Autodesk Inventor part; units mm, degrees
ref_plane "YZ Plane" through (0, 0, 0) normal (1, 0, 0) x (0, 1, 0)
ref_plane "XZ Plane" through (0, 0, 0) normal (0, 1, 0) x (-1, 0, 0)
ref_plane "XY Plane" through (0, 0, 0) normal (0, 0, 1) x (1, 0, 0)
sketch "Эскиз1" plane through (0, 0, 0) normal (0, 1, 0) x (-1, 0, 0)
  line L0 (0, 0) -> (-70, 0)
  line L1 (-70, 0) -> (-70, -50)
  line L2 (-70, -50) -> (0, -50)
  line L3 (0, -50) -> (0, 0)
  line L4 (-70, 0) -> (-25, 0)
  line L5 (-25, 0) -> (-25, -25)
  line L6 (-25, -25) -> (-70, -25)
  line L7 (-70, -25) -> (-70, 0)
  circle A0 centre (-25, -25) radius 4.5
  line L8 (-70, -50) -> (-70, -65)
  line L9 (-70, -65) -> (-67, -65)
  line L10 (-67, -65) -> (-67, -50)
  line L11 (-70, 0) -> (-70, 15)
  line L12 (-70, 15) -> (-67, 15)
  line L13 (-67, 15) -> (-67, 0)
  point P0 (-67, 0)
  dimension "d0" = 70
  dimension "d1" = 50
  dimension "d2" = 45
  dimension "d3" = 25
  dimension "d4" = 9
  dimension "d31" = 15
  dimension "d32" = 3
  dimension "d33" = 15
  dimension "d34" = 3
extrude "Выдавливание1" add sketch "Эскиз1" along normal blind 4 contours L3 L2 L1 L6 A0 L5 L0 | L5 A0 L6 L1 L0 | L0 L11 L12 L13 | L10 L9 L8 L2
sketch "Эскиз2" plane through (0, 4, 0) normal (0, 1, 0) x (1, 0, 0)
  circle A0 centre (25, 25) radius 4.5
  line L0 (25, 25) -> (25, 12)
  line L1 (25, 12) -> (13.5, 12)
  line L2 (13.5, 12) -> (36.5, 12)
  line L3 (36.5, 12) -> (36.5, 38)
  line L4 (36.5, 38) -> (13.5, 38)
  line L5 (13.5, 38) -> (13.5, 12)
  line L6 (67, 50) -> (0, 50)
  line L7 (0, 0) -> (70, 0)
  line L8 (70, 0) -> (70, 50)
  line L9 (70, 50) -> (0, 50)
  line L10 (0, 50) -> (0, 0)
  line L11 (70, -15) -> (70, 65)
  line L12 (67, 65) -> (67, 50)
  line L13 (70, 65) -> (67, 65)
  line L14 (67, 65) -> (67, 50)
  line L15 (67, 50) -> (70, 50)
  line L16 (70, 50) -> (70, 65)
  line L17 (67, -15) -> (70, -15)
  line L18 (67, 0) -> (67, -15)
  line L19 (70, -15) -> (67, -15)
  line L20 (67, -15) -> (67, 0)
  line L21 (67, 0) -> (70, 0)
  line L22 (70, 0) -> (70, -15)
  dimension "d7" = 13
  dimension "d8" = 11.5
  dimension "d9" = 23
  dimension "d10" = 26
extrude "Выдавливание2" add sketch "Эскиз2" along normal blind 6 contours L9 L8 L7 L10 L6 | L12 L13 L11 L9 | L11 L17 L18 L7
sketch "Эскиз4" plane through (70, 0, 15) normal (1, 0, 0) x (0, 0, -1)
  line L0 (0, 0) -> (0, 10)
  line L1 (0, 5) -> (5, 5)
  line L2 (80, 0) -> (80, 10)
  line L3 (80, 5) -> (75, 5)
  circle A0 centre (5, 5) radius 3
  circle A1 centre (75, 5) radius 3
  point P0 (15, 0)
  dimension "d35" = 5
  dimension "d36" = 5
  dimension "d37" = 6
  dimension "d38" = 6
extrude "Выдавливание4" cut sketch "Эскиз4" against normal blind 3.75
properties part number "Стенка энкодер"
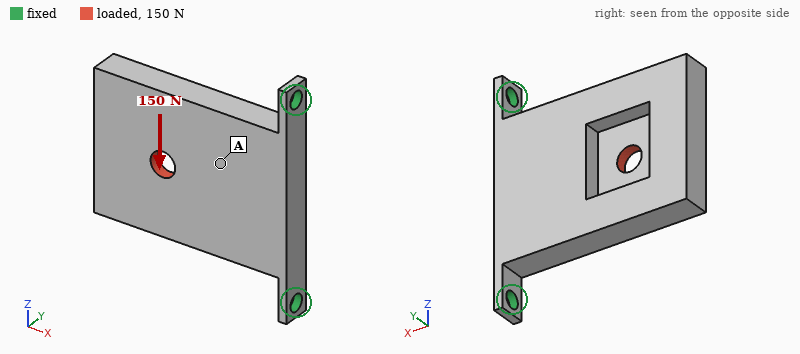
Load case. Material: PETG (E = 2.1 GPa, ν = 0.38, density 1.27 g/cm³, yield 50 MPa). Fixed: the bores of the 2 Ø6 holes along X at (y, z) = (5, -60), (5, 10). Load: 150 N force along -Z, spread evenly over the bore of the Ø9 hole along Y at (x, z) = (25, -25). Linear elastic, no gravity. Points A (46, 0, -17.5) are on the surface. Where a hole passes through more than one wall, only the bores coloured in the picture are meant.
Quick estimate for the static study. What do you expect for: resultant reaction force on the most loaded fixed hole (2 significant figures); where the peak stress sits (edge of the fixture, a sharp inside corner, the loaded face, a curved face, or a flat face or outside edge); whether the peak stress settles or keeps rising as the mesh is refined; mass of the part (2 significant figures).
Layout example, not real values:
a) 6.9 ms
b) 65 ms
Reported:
a) 140 N
b) edge of the fixture
c) keeps rising
d) 40 g
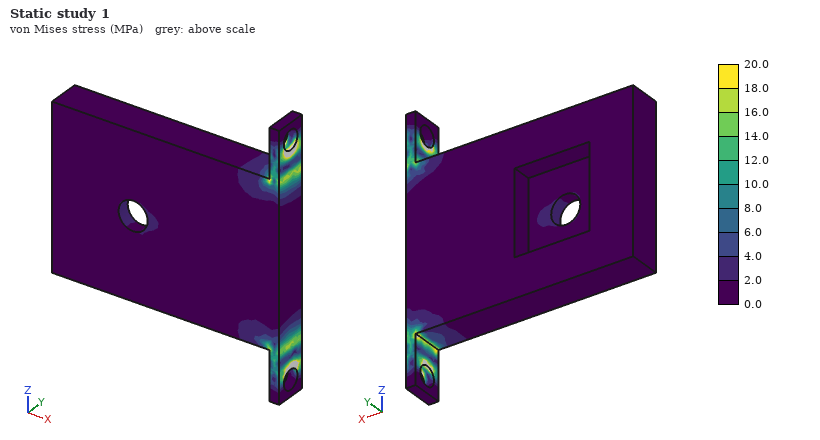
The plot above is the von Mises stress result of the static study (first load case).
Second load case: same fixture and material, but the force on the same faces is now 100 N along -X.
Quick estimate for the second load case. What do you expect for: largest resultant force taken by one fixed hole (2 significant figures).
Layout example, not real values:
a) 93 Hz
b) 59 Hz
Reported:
a) 59 N
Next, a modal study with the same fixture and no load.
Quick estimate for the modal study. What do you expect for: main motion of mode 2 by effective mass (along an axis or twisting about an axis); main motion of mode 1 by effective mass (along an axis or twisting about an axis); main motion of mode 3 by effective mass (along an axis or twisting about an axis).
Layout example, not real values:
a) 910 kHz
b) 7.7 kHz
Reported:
a) along Z
b) along Y
c) along X
